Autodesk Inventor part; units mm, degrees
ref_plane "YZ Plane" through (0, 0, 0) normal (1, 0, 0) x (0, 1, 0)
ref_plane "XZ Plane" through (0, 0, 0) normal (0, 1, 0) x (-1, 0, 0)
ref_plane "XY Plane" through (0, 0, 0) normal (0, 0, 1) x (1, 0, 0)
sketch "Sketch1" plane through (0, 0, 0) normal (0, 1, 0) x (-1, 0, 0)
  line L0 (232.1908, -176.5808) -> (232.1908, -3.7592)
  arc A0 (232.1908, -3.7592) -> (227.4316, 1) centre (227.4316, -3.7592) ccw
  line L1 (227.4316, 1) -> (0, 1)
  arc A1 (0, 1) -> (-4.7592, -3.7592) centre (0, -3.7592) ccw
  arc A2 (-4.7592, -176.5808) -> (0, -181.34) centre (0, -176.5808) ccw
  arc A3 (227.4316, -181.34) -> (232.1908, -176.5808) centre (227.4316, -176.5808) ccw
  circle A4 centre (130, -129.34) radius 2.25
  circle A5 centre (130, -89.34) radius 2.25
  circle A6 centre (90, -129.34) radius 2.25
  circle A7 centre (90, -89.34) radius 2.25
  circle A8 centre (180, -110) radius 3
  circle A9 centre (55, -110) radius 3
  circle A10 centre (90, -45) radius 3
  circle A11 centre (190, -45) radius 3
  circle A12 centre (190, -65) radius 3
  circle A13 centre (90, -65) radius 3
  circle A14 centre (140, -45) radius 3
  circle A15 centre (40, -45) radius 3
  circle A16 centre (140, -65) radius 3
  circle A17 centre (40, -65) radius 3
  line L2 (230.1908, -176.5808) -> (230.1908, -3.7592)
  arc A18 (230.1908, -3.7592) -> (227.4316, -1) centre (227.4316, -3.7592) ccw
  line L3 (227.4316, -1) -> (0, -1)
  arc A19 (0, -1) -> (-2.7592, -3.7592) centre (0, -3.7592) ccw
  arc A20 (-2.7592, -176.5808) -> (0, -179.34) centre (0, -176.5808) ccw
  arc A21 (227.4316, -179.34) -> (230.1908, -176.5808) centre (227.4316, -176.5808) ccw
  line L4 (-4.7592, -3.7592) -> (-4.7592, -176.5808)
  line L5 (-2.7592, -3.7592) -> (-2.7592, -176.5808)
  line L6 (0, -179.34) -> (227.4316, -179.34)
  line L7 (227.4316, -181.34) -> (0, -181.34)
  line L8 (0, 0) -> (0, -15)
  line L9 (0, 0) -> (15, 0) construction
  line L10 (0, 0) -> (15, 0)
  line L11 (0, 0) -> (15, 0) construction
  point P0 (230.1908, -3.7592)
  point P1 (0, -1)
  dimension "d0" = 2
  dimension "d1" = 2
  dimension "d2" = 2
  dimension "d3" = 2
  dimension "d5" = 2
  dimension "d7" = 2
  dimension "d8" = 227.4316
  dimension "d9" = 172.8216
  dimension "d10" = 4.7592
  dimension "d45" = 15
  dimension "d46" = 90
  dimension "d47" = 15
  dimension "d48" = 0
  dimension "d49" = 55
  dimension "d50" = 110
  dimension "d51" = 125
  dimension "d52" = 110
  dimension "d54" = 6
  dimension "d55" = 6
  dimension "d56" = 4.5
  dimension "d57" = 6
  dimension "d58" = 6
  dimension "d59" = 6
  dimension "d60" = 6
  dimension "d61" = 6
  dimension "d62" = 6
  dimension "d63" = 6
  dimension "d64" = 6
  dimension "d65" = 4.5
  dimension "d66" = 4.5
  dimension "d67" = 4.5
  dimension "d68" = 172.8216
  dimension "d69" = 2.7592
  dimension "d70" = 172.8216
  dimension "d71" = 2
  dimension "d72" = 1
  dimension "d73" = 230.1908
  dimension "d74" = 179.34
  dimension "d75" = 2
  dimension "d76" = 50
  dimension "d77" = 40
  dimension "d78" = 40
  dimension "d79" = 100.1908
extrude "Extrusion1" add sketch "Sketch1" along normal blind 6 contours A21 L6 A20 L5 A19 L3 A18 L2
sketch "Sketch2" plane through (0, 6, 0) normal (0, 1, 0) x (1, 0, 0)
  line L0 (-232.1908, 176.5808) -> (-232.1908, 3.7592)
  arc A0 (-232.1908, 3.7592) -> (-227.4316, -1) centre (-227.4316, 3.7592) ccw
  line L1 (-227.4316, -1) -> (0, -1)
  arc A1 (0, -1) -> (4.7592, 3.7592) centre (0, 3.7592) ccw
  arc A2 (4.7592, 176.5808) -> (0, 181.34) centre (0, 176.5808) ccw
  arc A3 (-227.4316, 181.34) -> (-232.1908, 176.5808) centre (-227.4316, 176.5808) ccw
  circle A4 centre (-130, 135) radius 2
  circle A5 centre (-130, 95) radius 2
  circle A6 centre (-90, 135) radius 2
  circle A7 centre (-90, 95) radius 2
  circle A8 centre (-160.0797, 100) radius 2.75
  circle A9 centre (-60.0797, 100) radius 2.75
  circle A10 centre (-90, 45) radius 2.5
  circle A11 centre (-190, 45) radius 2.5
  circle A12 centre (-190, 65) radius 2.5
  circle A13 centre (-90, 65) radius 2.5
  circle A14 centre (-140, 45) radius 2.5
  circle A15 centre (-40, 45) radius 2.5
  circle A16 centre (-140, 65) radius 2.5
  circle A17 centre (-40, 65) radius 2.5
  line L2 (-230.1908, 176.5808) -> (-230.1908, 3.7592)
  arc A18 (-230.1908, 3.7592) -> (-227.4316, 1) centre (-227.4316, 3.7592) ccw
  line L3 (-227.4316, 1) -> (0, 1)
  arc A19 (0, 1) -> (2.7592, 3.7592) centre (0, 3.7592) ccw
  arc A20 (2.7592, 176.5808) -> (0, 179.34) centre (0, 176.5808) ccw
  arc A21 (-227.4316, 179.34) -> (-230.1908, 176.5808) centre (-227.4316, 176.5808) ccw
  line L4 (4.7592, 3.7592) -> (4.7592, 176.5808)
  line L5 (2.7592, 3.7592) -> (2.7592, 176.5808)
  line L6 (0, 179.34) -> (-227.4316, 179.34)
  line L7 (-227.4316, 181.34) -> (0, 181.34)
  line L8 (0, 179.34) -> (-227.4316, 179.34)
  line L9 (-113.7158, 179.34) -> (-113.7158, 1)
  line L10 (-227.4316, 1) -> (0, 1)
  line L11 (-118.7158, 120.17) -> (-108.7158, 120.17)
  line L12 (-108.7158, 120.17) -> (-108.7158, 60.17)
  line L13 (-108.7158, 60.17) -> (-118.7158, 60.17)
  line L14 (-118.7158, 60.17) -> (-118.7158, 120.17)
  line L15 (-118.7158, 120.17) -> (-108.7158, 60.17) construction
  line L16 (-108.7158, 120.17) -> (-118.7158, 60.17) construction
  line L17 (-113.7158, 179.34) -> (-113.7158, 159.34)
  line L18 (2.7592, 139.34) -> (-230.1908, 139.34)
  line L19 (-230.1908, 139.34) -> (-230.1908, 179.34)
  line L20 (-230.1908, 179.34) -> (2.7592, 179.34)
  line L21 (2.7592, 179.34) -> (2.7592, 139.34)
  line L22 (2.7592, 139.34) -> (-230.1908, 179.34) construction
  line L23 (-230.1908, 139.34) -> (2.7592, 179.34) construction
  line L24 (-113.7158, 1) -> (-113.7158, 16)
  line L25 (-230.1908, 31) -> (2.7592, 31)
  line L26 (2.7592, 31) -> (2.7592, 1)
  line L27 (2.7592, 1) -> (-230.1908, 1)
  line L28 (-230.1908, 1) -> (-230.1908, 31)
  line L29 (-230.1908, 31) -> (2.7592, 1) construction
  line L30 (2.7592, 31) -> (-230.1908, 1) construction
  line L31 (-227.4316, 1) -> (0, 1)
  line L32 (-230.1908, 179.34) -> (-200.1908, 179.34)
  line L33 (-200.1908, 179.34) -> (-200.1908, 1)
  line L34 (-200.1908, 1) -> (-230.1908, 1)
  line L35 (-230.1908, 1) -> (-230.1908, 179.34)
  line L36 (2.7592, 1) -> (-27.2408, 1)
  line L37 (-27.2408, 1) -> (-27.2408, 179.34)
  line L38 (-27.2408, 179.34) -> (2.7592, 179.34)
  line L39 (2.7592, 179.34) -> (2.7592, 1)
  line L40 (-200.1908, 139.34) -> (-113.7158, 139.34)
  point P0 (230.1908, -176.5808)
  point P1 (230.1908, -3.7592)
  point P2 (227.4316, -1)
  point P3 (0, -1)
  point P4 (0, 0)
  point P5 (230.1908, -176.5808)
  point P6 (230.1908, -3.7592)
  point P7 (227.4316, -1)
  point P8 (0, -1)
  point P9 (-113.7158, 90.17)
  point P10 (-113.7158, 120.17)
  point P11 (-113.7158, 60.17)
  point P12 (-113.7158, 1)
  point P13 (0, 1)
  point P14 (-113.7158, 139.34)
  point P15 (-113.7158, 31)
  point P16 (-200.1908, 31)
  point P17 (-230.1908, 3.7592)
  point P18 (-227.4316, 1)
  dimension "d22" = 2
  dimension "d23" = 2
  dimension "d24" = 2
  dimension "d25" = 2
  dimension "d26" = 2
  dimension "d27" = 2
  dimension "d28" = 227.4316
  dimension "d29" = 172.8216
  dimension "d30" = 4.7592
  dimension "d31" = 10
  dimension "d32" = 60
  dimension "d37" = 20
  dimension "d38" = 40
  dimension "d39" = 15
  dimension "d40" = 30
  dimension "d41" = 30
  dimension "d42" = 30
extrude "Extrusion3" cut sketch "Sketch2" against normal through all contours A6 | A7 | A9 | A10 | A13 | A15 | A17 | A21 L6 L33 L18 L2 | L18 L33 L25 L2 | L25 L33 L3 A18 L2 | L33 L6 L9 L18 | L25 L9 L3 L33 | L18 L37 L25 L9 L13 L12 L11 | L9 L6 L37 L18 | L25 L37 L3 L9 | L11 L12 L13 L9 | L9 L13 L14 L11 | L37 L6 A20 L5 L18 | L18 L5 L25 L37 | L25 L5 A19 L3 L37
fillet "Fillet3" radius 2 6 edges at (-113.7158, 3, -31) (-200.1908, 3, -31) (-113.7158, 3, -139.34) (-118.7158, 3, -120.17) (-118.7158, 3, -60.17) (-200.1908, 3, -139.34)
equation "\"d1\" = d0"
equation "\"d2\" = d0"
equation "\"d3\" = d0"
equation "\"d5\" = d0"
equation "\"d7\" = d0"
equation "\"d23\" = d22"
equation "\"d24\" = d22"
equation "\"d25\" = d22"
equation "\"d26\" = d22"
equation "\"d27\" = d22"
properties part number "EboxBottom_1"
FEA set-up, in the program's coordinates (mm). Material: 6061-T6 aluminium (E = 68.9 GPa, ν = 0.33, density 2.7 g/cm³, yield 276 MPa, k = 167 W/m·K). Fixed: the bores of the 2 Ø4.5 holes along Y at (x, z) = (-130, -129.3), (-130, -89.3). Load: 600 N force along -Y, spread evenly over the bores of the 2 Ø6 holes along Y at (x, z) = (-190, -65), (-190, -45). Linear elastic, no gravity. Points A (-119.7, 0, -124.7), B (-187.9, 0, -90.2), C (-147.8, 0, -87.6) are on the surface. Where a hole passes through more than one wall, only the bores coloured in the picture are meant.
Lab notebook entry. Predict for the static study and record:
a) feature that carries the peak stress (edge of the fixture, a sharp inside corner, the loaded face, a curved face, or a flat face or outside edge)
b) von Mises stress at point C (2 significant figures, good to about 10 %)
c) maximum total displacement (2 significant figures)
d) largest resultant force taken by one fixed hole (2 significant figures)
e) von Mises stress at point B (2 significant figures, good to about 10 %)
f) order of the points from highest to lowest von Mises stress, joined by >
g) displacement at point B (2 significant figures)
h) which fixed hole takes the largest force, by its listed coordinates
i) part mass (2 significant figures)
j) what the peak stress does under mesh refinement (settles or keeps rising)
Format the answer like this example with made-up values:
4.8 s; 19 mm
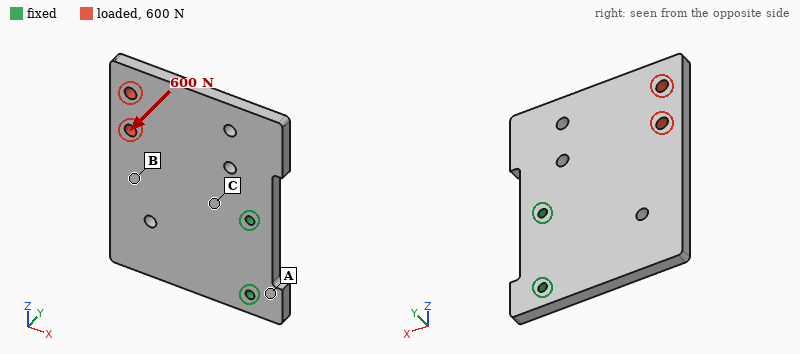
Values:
edge of the fixture; 67 MPa; 1.2 mm; 920 N; 33 MPa; C > B > A; 0.52 mm; (-130, -89.3); 140 g; keeps rising
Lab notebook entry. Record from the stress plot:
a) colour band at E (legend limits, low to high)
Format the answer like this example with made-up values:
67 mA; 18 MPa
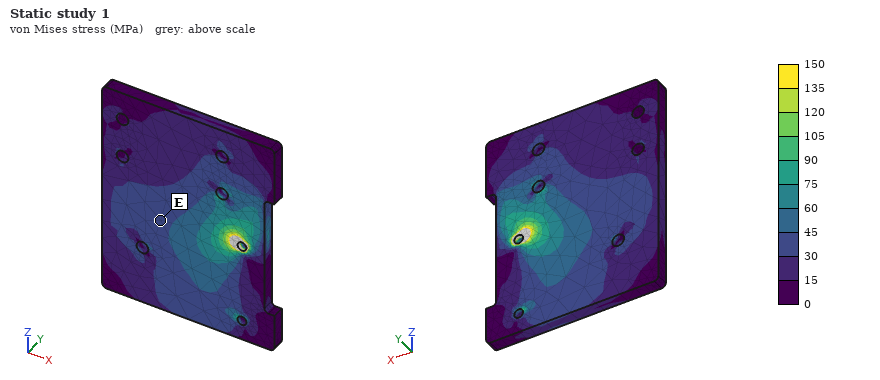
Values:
30 to 45 MPa
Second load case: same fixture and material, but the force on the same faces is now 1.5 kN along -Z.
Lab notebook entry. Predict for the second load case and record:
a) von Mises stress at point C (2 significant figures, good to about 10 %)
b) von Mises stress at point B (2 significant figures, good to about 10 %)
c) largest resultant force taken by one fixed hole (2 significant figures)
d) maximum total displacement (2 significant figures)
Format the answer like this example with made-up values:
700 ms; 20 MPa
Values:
10 MPa; 7.2 MPa; 2.3 kN; 50 µm
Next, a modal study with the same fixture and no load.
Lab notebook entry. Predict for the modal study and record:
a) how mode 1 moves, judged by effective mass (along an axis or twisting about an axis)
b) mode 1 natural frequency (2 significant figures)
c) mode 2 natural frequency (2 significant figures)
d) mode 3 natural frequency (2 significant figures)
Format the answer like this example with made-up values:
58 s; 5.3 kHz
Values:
along Y; 720 Hz; 1100 Hz; 2100 Hz
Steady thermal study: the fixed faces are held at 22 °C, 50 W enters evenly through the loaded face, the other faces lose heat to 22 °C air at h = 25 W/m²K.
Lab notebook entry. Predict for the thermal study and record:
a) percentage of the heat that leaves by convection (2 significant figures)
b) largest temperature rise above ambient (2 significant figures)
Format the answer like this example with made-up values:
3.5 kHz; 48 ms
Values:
22 %; 56 K
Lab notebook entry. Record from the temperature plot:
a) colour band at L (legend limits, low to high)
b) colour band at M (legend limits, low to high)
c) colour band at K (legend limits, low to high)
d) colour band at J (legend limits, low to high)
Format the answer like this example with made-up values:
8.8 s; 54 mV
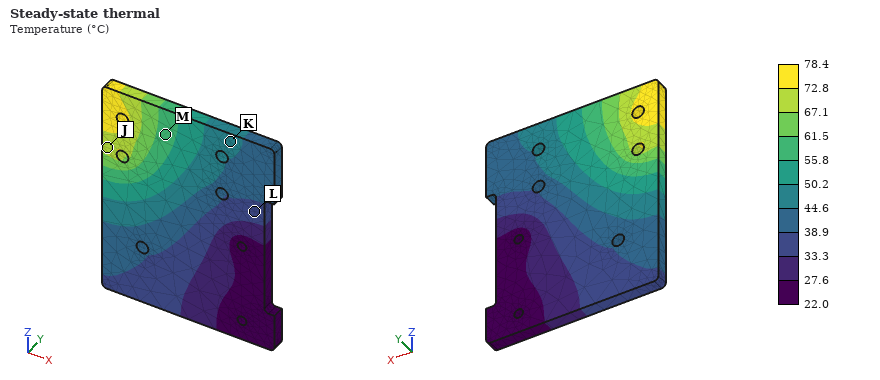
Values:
33.3 to 38.9 °C; 55.8 to 61.5 °C; 44.6 to 50.2 °C; 67.1 to 72.8 °C
